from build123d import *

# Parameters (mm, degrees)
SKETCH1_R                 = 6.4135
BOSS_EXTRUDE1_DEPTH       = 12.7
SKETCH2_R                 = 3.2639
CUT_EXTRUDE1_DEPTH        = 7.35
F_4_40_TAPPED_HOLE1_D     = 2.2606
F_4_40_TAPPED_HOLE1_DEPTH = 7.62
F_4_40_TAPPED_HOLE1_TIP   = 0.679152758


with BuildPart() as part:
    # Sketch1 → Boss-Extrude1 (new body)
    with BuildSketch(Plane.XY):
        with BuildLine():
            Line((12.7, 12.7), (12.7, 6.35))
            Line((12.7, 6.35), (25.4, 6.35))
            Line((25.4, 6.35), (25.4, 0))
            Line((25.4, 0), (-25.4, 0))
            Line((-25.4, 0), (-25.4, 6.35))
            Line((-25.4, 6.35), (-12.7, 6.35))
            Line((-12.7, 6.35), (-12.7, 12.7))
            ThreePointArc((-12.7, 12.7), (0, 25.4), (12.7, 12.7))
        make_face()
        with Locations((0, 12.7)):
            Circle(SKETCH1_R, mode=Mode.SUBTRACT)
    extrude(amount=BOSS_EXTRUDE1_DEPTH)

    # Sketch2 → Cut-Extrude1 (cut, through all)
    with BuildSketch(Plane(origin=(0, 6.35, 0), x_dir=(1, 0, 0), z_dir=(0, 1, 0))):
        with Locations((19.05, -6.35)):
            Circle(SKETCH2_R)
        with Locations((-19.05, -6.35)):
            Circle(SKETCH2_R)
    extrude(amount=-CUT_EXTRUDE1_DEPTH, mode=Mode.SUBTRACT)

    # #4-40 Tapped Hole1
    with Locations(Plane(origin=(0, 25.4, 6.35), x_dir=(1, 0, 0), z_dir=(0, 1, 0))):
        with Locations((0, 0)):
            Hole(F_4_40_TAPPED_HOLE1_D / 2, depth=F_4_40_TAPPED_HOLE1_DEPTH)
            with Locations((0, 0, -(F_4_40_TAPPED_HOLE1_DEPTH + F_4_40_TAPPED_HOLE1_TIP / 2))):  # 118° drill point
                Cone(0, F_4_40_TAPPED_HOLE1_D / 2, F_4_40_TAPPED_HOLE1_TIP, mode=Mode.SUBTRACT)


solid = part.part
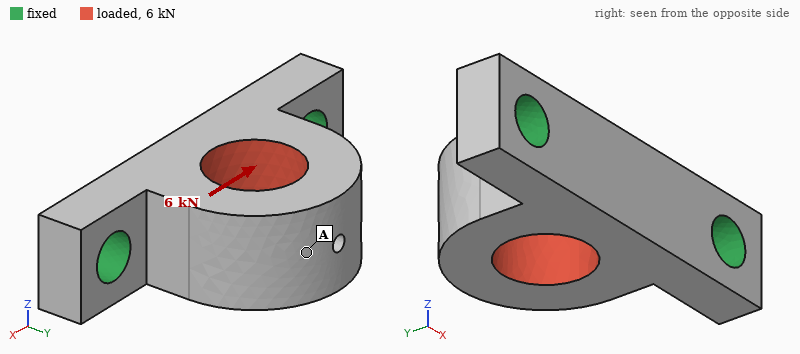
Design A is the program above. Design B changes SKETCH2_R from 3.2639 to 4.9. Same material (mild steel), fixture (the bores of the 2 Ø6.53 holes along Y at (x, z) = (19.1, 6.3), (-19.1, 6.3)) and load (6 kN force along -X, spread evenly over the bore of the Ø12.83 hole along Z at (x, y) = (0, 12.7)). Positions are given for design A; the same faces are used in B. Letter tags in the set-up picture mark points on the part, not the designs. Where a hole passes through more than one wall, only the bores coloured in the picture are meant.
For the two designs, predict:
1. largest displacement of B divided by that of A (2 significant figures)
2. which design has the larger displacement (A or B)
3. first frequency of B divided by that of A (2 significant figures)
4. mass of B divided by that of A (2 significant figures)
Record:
0.90
A
1.2
0.93
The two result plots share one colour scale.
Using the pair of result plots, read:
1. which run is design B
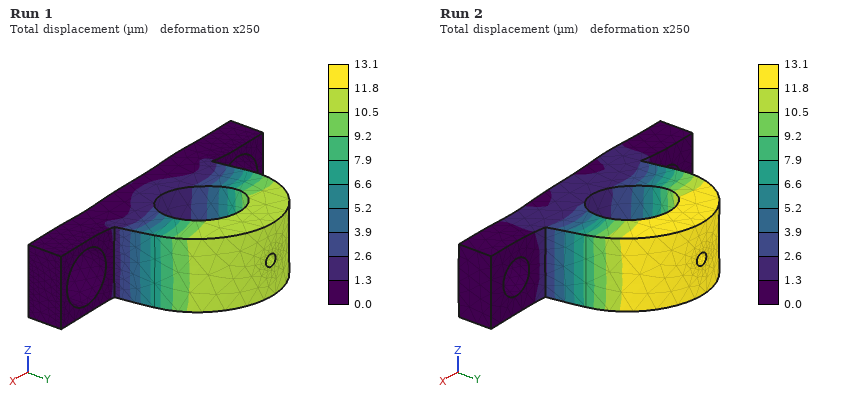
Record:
Run 1
